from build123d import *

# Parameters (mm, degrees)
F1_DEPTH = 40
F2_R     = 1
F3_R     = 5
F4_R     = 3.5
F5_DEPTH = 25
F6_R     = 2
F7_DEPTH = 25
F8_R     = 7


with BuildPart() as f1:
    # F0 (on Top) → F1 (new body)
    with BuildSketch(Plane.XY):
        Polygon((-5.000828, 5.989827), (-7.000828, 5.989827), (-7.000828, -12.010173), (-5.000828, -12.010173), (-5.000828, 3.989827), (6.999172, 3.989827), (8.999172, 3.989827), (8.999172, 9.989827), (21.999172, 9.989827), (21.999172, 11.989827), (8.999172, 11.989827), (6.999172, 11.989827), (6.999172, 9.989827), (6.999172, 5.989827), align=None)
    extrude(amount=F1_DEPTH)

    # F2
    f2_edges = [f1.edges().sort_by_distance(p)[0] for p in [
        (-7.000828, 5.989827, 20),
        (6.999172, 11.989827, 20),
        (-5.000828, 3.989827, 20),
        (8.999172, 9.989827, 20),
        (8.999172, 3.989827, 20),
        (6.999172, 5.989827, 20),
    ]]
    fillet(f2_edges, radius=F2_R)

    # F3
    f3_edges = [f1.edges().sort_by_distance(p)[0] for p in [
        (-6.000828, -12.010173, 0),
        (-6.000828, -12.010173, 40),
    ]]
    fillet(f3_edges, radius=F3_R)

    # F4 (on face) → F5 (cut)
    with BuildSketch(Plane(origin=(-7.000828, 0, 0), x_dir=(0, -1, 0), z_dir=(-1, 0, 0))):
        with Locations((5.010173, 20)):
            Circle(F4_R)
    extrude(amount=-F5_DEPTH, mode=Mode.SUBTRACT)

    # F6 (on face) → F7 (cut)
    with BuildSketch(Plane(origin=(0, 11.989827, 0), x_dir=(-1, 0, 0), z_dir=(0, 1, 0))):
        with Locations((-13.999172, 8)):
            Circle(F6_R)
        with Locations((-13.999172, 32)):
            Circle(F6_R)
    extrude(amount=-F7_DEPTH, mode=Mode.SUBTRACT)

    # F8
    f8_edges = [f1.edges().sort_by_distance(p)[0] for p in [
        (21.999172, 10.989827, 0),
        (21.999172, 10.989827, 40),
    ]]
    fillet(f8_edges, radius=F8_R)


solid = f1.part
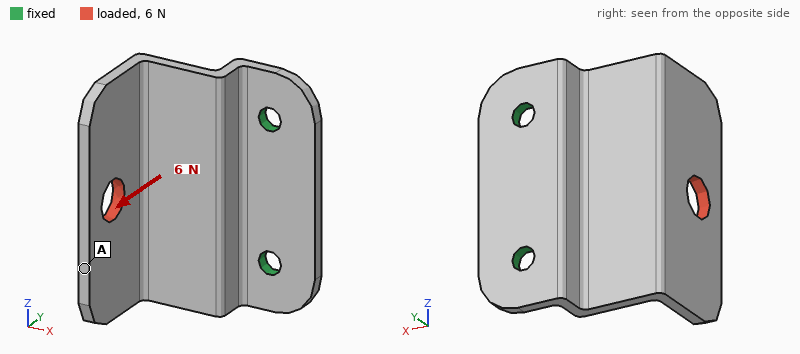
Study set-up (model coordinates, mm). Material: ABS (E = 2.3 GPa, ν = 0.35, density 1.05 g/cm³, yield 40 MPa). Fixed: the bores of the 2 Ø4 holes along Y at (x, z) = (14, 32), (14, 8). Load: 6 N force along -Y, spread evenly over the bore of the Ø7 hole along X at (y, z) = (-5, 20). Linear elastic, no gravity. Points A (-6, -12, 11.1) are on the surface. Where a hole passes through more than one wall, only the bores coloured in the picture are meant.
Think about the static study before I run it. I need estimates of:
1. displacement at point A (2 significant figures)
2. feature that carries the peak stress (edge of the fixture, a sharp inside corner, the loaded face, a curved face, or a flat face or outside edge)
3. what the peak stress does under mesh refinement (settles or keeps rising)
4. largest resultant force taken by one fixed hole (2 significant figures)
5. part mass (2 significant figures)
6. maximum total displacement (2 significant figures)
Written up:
0.50 mm
edge of the fixture
keeps rising
3.3 N
4.1 g
0.52 mm
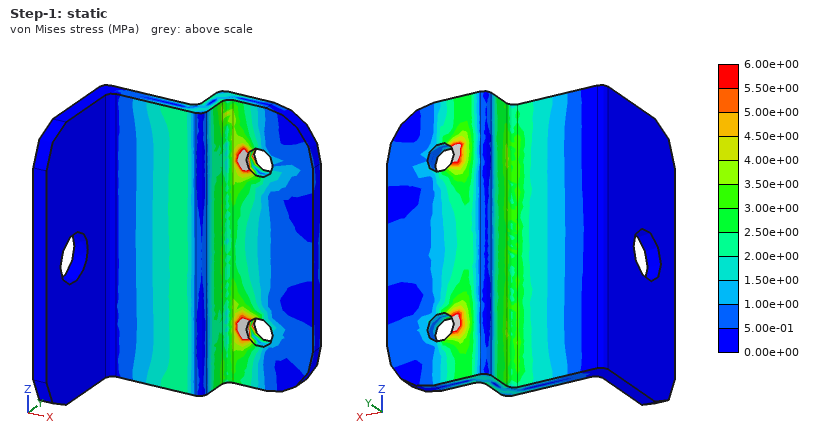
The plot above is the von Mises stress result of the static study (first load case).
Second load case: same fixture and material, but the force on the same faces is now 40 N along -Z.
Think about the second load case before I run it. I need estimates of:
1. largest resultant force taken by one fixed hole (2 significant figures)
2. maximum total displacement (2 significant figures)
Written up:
44 N
0.62 mm
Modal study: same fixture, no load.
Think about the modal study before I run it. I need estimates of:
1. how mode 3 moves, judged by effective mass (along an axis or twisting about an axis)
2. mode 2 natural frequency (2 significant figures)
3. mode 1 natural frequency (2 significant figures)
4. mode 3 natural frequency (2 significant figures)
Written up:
along Y
900 Hz
430 Hz
1700 Hz
